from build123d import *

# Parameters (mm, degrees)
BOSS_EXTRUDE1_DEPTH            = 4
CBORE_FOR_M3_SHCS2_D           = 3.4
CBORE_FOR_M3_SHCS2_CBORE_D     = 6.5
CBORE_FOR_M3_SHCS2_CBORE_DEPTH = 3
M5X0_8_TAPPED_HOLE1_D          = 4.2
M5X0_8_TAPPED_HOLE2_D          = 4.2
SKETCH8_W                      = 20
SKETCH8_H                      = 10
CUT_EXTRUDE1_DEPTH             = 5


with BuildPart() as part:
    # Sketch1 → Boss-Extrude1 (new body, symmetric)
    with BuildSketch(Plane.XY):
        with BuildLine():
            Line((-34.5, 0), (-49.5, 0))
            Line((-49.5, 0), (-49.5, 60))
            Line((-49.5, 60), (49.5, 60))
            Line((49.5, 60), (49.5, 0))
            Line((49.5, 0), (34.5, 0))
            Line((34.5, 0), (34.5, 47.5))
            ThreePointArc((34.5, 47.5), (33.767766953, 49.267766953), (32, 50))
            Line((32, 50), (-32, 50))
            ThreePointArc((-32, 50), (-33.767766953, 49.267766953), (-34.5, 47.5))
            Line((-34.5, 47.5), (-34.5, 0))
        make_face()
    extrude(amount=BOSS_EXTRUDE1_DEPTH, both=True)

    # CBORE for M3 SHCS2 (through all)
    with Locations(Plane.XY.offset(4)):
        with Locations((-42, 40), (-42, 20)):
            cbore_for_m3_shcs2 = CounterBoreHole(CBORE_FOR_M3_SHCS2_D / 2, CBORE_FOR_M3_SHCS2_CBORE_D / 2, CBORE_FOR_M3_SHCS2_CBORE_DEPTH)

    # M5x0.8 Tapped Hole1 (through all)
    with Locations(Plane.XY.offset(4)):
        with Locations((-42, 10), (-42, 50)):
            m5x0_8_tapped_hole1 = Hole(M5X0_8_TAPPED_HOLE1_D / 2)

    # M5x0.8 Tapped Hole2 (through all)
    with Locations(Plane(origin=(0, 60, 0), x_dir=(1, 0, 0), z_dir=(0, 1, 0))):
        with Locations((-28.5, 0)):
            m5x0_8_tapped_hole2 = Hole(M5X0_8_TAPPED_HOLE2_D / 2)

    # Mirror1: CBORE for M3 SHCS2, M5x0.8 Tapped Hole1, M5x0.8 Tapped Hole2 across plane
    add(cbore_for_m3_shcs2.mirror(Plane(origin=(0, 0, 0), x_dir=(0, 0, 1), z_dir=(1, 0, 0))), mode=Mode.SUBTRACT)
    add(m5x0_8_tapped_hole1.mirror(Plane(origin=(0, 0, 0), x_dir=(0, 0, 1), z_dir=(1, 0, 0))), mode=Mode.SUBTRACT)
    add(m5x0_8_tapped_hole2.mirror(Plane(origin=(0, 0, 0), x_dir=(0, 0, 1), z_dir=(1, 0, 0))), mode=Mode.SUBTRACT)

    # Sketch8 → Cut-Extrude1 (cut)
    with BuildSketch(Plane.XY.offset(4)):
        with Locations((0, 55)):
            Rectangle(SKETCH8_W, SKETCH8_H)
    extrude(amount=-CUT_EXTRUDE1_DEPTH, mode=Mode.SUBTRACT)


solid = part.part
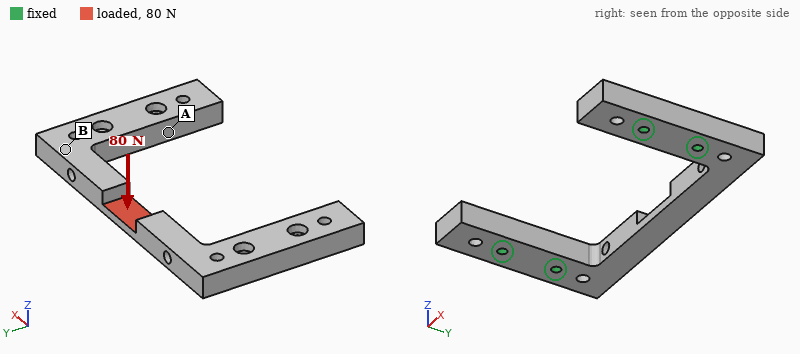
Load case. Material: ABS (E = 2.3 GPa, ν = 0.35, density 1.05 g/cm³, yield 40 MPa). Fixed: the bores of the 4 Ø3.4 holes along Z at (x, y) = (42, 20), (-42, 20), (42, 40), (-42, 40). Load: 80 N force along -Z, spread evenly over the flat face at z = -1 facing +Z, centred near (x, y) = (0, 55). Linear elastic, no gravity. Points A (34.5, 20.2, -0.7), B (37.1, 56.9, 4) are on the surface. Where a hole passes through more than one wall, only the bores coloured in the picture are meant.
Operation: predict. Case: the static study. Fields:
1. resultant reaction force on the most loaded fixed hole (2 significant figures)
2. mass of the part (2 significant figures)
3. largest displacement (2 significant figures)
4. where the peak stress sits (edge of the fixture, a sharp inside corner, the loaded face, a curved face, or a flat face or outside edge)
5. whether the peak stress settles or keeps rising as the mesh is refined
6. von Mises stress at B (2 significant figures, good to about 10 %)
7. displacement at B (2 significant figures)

100 N
19 g
1.1 mm
edge of the fixture
keeps rising
6.7 MPa
0.20 mm
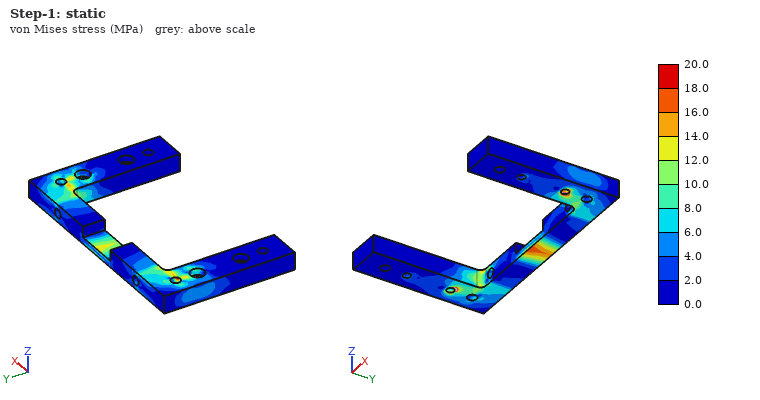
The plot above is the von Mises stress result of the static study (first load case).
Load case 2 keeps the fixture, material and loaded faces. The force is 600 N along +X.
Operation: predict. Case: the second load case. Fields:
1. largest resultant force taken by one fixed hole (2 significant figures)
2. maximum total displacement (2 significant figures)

420 N
0.38 mm
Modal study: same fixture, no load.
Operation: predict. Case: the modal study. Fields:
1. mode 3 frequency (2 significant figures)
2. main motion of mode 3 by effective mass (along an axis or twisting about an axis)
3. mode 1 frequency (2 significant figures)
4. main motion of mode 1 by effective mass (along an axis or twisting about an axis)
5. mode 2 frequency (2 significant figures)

2100 Hz
along Y
1000 Hz
along Z
2000 Hz
